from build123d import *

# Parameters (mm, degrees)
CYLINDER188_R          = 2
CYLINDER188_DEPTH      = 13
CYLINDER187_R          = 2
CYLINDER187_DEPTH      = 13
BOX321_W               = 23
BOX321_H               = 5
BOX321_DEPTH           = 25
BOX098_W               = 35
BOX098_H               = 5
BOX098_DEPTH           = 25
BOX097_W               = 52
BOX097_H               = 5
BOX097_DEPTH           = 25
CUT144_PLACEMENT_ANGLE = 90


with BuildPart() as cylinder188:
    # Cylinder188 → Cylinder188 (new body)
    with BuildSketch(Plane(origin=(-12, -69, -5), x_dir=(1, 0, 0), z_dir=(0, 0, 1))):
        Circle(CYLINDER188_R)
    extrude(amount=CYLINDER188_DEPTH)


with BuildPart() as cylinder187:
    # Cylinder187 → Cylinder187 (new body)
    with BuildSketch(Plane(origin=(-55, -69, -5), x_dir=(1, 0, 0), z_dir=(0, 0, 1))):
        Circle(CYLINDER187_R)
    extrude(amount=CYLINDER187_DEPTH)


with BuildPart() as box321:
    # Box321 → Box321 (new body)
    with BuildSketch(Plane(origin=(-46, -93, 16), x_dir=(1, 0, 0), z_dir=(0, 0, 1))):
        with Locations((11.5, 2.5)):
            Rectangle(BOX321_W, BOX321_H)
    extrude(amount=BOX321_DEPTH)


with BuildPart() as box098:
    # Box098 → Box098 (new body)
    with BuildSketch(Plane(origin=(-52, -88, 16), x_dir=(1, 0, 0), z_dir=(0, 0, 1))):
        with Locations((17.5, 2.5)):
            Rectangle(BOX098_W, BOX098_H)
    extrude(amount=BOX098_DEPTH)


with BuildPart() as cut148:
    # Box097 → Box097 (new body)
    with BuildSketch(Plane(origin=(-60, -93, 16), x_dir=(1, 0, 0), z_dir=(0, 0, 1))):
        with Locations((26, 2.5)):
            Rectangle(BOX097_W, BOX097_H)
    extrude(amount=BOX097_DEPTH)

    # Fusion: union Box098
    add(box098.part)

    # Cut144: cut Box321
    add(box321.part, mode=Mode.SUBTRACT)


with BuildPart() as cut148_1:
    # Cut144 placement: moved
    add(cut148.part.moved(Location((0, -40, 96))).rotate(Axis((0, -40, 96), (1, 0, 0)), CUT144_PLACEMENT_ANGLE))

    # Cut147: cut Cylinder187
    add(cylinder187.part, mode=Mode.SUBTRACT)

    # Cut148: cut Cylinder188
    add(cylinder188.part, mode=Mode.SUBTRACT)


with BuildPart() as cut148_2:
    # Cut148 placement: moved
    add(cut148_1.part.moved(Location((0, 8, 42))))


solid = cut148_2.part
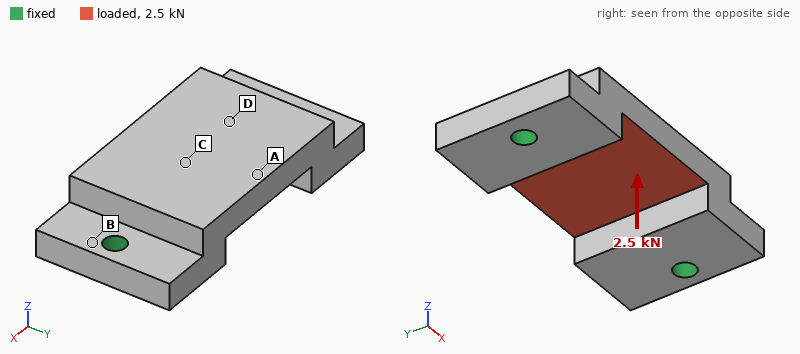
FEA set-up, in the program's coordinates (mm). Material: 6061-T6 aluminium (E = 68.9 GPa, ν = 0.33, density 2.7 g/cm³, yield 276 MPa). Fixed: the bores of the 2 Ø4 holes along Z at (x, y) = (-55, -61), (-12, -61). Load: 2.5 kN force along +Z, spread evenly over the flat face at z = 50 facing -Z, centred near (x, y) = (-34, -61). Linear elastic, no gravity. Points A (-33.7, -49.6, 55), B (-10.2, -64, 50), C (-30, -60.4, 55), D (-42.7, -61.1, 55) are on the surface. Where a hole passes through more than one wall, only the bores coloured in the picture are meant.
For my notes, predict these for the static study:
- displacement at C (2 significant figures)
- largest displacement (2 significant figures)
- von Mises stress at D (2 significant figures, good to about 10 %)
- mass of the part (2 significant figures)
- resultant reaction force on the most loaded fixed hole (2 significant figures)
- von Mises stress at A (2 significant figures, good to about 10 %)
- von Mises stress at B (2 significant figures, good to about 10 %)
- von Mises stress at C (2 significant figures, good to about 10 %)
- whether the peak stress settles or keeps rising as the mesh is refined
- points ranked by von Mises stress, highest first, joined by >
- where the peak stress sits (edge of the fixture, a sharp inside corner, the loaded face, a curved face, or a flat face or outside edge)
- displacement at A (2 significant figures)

28 µm
37 µm
28 MPa
21 g
2.2 kN
60 MPa
12 MPa
50 MPa
keeps rising
A > C > D > B
edge of the fixture
35 µm
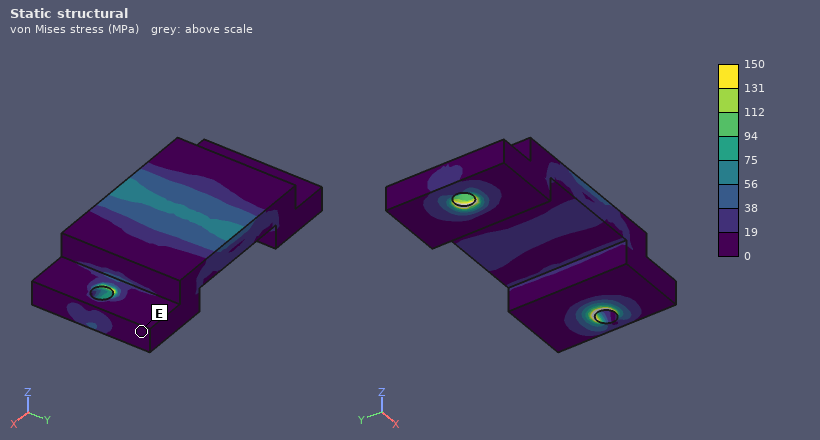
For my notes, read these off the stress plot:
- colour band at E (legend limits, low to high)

0 to 19 MPa
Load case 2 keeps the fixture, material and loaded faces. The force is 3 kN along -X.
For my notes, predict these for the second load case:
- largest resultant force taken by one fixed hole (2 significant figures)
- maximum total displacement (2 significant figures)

1.6 kN
12 µm
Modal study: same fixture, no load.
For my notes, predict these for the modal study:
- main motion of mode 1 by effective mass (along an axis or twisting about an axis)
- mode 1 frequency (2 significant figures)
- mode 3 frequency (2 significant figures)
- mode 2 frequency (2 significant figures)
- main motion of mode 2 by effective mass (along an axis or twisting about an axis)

along Y
11 kHz
20 kHz
16 kHz
along Z
